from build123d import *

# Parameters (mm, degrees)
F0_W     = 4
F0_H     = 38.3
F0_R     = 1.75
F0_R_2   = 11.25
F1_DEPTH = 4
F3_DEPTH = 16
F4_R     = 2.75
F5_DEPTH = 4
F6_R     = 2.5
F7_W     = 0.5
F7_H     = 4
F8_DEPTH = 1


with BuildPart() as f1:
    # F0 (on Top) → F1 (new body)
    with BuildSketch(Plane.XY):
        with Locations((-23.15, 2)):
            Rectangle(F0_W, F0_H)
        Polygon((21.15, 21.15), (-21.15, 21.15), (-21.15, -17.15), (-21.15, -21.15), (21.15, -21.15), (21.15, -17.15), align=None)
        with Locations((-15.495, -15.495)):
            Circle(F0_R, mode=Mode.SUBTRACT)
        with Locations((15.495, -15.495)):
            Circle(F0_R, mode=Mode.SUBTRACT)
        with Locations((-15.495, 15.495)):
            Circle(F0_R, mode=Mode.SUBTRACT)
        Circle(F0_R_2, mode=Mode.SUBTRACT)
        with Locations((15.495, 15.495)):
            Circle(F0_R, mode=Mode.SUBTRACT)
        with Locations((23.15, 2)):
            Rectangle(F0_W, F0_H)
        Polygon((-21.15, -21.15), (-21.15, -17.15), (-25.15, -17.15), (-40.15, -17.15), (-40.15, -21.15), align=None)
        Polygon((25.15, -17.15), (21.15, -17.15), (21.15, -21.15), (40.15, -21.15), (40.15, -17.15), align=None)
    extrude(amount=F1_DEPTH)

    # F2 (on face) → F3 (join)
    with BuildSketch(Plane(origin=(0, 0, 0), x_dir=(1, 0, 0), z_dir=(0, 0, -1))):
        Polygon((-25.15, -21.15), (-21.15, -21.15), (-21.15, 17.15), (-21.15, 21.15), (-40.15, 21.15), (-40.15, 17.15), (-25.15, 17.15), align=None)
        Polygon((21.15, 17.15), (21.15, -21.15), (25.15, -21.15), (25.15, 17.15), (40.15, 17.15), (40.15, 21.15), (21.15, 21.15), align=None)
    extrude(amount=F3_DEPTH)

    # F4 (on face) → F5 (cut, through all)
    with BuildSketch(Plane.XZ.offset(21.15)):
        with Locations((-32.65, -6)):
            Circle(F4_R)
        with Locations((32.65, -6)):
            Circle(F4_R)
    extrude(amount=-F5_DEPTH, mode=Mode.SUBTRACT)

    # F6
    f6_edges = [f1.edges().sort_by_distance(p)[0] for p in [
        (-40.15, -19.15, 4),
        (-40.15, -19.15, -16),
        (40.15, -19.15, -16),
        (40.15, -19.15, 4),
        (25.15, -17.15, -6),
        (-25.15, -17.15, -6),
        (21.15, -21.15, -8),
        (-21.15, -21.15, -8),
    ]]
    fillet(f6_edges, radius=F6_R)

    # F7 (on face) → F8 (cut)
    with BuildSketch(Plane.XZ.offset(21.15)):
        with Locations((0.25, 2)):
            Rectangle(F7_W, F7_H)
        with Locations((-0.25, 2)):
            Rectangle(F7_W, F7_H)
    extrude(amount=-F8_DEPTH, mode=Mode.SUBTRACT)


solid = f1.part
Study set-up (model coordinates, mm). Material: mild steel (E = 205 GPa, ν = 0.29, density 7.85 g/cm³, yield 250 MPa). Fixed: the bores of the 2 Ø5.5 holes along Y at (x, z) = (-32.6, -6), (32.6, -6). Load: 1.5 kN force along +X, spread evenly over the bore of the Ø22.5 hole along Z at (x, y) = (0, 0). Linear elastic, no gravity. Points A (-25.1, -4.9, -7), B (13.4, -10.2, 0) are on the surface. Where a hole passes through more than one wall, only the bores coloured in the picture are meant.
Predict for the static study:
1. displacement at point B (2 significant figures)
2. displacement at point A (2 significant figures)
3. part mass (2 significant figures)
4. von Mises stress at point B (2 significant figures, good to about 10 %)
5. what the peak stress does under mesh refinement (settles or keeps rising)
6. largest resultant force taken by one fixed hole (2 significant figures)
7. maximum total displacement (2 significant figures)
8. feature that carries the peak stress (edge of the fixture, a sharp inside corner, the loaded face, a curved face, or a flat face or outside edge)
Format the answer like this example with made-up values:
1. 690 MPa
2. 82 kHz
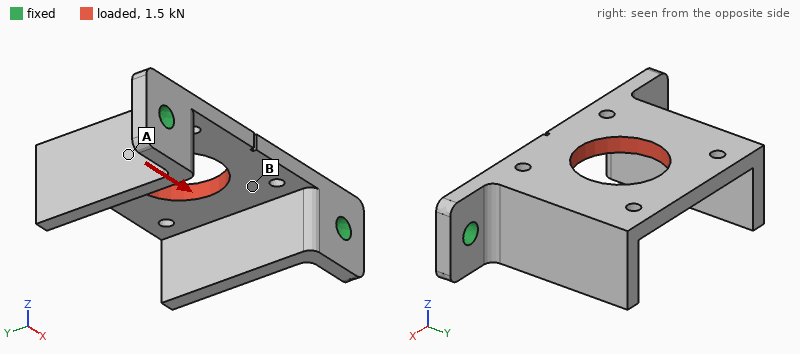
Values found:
1. 6.2 µm
2. 7.4 µm
3. 110 g
4. 17 MPa
5. keeps rising
6. 900 N
7. 21 µm
8. edge of the fixture
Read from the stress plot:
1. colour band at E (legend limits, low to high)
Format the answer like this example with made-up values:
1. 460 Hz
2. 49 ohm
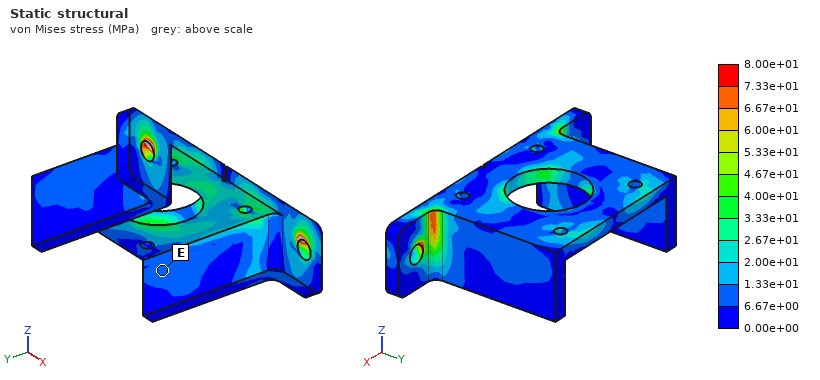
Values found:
1. 6.67e+00 to 1.33e+01 MPa
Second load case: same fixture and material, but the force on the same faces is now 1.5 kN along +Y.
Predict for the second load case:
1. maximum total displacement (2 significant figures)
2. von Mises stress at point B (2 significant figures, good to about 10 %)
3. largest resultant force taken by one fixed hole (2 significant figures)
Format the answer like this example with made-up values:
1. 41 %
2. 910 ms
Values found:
1. 45 µm
2. 12 MPa
3. 820 N
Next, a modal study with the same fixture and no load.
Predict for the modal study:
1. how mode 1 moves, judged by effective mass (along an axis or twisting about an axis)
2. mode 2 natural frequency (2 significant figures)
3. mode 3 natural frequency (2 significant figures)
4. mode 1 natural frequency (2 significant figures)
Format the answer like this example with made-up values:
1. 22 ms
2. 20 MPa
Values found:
1. along Z
2. 3000 Hz
3. 5400 Hz
4. 2200 Hz
